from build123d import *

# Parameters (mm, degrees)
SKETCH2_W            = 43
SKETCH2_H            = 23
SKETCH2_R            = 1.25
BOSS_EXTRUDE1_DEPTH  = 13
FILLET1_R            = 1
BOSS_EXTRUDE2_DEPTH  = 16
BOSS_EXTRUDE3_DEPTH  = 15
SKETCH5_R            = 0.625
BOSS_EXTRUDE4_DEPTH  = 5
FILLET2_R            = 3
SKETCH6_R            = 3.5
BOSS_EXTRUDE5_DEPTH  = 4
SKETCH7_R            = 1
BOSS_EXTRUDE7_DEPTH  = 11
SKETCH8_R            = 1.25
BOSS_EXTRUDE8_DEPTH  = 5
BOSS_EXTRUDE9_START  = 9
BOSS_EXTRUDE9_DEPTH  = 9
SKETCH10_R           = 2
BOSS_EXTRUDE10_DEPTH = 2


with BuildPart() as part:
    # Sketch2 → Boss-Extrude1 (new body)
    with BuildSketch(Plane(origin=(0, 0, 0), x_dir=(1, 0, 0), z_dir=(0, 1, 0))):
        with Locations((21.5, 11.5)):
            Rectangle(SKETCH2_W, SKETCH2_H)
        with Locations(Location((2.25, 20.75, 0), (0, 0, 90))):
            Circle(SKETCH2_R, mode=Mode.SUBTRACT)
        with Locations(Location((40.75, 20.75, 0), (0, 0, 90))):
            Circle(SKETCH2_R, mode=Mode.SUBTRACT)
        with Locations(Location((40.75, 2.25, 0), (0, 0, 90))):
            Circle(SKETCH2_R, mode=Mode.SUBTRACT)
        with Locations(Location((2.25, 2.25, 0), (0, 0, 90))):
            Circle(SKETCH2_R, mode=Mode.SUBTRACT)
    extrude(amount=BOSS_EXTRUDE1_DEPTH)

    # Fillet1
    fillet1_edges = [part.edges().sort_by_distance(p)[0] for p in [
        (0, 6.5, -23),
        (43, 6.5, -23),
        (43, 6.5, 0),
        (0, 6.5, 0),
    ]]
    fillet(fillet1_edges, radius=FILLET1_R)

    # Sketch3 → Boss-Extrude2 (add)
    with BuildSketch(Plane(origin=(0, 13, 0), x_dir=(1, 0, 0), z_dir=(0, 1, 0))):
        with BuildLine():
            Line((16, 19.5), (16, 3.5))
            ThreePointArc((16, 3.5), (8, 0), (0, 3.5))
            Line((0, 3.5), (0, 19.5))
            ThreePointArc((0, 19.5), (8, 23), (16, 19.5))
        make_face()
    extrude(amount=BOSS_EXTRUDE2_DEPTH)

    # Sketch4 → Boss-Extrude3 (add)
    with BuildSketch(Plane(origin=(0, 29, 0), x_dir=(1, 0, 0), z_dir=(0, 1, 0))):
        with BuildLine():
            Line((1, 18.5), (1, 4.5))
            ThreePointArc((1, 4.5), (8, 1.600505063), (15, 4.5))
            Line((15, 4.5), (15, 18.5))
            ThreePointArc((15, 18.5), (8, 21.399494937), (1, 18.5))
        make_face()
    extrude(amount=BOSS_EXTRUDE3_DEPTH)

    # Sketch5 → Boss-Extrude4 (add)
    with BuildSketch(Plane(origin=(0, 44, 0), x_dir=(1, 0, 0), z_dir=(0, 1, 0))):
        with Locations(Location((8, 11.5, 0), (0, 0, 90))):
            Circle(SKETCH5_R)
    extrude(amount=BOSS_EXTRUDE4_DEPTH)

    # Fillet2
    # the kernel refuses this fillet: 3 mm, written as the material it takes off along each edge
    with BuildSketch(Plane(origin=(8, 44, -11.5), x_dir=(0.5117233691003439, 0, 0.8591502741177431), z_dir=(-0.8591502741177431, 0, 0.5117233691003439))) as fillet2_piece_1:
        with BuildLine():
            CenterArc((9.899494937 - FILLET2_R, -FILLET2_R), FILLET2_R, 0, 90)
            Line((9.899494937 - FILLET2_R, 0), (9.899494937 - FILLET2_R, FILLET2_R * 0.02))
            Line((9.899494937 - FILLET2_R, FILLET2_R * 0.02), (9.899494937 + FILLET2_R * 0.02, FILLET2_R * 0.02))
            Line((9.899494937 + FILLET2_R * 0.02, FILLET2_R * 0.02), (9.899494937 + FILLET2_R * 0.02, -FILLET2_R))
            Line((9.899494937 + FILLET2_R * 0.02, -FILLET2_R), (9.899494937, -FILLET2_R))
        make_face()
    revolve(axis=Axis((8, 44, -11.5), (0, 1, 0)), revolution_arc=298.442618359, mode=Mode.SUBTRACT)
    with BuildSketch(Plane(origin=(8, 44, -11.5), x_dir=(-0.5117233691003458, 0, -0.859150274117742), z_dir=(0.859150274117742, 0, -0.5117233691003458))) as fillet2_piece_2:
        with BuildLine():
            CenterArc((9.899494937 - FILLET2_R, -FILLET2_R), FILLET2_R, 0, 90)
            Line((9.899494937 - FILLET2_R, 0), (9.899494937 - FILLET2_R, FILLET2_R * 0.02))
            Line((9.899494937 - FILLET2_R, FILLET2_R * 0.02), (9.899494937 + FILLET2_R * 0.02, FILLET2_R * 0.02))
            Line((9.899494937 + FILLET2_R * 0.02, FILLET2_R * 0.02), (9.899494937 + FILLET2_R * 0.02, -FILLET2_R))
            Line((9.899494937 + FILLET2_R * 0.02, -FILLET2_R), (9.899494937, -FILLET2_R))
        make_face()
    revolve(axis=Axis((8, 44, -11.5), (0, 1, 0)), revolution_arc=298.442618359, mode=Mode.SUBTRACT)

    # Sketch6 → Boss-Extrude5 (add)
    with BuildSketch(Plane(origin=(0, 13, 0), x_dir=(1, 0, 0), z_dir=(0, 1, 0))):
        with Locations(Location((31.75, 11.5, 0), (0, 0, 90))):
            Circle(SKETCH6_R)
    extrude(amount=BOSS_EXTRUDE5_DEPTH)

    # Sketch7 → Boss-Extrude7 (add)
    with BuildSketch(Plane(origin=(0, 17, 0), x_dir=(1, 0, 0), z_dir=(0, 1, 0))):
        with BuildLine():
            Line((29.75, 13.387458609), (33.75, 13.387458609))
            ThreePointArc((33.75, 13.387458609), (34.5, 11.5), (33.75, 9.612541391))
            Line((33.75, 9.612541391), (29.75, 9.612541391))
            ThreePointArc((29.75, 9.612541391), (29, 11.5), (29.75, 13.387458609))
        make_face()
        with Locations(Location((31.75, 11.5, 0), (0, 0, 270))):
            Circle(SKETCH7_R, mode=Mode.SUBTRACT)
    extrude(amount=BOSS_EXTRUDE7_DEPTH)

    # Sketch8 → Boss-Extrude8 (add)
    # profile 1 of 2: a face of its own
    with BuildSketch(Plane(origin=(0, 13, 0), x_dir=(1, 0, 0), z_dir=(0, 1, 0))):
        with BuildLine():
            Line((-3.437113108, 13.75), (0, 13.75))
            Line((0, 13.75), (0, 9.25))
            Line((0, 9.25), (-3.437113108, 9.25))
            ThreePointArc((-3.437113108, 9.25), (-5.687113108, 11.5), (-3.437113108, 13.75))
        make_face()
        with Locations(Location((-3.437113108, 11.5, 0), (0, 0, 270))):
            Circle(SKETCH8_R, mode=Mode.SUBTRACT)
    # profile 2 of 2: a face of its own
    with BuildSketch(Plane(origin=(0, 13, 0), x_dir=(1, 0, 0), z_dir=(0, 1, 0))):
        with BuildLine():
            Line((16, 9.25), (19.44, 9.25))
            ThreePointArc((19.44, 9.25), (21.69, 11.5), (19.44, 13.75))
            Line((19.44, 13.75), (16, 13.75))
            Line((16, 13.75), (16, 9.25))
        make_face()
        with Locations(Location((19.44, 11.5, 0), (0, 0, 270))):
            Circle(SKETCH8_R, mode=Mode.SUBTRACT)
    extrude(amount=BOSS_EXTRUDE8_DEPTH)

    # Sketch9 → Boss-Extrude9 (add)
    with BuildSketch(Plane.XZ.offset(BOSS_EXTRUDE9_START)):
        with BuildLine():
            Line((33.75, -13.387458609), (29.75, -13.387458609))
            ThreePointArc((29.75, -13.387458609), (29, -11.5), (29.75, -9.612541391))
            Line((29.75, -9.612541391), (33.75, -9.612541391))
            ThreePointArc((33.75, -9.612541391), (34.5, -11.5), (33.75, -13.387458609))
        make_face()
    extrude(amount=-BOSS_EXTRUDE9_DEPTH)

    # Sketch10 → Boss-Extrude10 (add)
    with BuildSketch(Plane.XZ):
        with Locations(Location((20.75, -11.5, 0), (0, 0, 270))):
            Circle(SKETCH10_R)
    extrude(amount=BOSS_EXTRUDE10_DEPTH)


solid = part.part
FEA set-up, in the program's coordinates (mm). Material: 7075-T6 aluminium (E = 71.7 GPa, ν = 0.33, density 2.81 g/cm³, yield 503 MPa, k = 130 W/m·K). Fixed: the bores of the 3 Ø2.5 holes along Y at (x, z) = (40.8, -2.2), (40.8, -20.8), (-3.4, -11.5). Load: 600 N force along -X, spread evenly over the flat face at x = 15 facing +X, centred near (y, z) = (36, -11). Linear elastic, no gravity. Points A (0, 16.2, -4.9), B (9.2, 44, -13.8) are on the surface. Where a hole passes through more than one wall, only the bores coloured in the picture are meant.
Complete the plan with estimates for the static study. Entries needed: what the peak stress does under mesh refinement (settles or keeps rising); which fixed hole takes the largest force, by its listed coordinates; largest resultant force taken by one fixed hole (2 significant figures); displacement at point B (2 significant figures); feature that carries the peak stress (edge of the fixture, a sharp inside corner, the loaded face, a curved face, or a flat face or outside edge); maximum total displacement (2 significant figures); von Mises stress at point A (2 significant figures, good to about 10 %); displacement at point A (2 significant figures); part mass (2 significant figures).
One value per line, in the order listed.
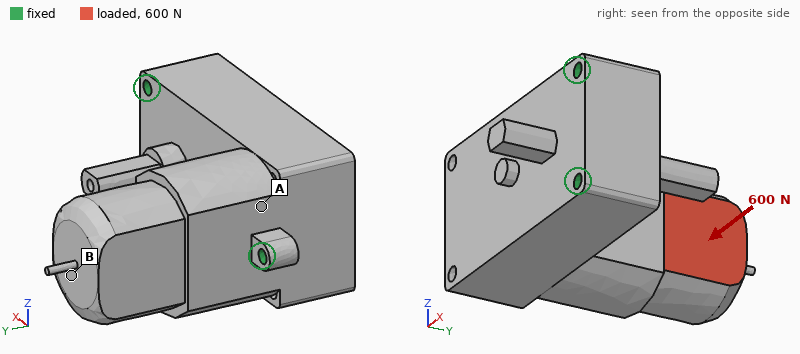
keeps rising
(-3.4, -11.5)
700 N
18 µm
edge of the fixture
21 µm
10 MPa
3.3 µm
63 g
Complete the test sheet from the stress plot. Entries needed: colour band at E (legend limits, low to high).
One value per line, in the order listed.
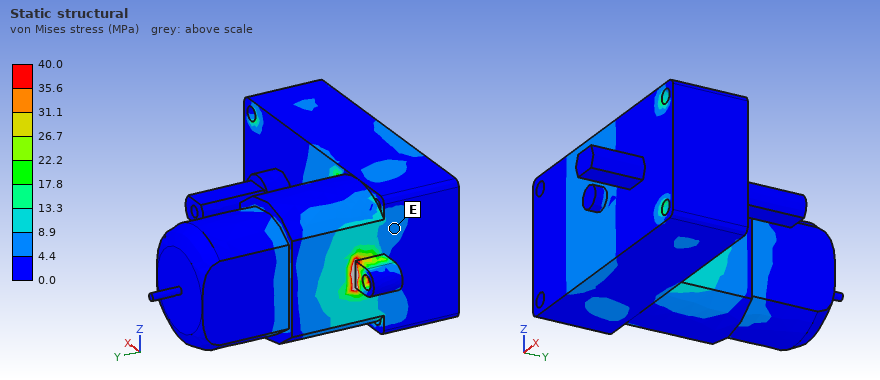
4.4 to 8.9 MPa
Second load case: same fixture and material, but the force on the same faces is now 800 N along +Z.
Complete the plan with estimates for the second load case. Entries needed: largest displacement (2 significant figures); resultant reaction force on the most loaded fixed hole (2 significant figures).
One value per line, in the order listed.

72 µm
800 N
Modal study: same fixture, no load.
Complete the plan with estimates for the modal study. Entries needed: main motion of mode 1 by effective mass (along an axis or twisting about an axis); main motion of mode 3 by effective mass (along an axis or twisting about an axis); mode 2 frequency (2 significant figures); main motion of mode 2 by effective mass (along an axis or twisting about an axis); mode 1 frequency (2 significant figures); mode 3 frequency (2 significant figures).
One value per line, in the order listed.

along Z
along Y
9200 Hz
along X
5200 Hz
10 kHz
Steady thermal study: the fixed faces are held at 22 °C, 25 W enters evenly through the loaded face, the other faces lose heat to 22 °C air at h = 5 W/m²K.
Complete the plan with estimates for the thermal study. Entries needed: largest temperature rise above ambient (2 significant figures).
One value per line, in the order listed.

31 K
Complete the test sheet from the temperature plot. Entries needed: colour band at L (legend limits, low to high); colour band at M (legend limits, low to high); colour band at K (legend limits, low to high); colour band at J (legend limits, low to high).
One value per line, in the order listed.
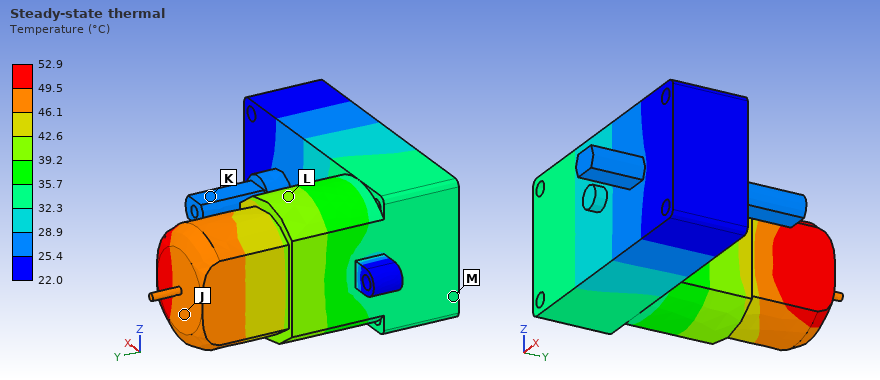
39.2 to 42.6 °C
32.3 to 35.7 °C
25.4 to 28.9 °C
46.1 to 49.5 °C
